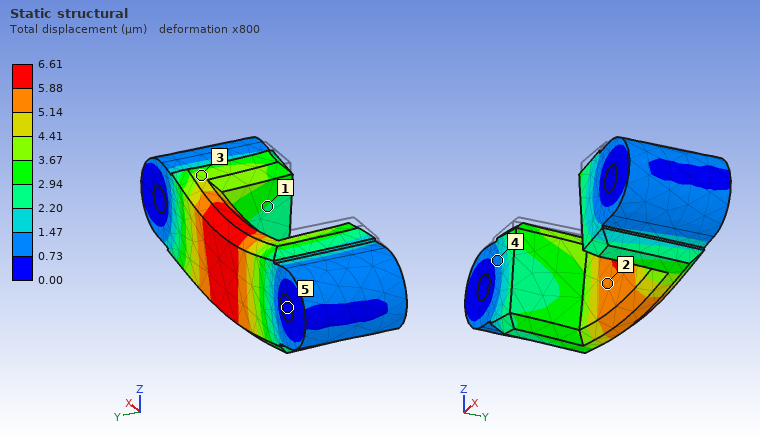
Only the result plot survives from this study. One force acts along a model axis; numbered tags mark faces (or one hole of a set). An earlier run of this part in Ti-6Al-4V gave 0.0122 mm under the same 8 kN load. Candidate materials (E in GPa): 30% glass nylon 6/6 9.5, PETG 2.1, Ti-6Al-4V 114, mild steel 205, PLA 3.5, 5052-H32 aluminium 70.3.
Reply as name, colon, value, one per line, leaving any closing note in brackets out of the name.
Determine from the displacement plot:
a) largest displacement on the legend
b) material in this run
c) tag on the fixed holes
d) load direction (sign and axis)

largest displacement on the legend: 6.61 µm
material in this run: mild steel
tag on the fixed holes: 5
load direction: -Z
